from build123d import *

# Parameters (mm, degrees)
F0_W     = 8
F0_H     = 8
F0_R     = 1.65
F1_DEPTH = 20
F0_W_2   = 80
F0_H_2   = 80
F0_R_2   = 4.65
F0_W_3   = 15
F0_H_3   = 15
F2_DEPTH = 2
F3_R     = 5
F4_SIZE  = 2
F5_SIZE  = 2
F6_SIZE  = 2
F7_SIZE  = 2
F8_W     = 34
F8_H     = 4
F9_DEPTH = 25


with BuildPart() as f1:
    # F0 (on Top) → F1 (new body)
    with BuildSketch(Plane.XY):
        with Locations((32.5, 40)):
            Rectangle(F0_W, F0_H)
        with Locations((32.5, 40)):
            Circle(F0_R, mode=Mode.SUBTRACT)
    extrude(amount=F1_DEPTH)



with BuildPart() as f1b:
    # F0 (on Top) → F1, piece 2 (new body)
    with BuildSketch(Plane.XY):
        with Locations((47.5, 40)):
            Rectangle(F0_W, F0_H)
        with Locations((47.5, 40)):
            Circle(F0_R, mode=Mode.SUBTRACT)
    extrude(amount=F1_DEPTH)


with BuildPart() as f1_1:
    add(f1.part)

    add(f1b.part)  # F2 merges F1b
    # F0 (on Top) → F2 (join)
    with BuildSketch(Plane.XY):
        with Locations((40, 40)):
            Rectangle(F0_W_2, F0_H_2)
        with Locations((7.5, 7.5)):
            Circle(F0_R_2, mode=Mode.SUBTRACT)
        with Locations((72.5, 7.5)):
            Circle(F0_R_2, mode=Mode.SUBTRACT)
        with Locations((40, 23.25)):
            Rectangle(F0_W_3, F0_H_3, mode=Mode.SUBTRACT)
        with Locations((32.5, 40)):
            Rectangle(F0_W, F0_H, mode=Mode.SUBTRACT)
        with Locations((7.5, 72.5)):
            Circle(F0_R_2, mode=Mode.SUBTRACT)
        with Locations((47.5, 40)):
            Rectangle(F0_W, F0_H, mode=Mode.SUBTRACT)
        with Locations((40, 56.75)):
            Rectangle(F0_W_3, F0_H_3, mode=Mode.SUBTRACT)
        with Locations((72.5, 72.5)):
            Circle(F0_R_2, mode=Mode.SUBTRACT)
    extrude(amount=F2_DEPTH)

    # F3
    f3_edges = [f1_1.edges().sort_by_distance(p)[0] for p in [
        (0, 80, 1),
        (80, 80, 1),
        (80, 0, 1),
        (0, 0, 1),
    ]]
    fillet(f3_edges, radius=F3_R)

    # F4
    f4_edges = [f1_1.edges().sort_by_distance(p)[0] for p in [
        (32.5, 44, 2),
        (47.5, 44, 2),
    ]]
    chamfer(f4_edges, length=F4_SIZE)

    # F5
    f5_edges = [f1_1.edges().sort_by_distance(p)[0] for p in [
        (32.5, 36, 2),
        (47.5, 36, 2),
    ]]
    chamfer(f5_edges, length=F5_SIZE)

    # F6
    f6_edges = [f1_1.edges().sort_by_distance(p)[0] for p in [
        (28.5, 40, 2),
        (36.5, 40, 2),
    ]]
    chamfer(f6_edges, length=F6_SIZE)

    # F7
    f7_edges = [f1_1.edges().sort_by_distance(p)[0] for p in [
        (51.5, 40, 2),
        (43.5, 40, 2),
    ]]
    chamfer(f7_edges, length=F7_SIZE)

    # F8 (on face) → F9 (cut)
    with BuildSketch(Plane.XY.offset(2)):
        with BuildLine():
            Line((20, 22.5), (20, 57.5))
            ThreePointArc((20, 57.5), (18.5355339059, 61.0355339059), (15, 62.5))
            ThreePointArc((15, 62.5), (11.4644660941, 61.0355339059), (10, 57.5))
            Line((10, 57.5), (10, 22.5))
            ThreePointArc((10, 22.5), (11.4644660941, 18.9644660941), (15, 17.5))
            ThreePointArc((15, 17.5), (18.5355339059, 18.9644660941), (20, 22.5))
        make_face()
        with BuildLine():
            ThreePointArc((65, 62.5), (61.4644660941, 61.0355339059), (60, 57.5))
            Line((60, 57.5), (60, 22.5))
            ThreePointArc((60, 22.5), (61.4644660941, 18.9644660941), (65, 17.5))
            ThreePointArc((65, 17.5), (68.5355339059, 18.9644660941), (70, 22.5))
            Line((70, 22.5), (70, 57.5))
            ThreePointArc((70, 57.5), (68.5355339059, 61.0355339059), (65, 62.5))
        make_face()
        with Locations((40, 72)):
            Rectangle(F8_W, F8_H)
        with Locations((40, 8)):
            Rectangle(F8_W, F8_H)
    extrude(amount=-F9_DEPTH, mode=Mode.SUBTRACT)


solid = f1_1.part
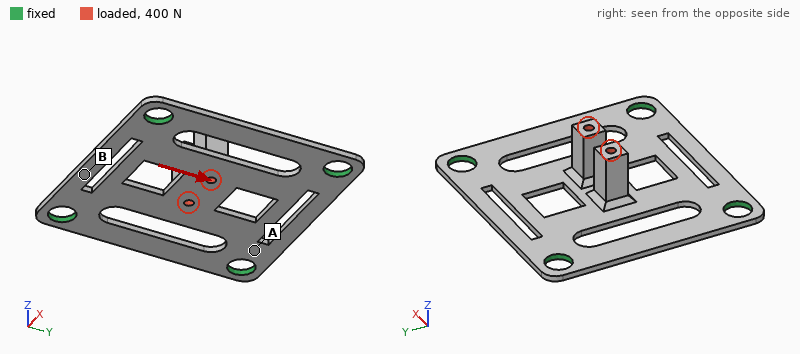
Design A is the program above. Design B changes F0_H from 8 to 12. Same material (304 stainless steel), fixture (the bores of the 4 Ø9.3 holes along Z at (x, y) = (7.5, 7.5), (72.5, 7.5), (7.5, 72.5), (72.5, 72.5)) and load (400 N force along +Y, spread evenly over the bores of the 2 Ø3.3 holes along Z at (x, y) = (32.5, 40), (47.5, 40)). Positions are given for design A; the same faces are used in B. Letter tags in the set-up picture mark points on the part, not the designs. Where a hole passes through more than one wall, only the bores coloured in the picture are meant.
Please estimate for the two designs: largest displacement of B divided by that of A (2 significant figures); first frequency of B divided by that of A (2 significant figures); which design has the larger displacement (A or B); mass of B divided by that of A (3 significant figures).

0.83
0.93
A
1.11
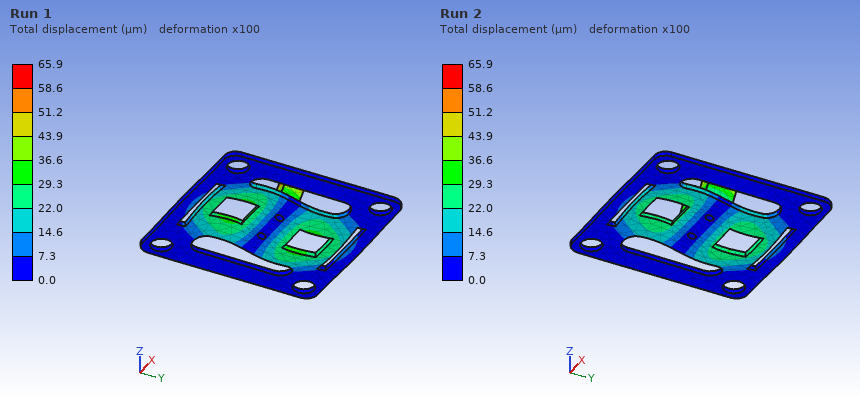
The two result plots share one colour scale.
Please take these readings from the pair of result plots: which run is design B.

Run 2
